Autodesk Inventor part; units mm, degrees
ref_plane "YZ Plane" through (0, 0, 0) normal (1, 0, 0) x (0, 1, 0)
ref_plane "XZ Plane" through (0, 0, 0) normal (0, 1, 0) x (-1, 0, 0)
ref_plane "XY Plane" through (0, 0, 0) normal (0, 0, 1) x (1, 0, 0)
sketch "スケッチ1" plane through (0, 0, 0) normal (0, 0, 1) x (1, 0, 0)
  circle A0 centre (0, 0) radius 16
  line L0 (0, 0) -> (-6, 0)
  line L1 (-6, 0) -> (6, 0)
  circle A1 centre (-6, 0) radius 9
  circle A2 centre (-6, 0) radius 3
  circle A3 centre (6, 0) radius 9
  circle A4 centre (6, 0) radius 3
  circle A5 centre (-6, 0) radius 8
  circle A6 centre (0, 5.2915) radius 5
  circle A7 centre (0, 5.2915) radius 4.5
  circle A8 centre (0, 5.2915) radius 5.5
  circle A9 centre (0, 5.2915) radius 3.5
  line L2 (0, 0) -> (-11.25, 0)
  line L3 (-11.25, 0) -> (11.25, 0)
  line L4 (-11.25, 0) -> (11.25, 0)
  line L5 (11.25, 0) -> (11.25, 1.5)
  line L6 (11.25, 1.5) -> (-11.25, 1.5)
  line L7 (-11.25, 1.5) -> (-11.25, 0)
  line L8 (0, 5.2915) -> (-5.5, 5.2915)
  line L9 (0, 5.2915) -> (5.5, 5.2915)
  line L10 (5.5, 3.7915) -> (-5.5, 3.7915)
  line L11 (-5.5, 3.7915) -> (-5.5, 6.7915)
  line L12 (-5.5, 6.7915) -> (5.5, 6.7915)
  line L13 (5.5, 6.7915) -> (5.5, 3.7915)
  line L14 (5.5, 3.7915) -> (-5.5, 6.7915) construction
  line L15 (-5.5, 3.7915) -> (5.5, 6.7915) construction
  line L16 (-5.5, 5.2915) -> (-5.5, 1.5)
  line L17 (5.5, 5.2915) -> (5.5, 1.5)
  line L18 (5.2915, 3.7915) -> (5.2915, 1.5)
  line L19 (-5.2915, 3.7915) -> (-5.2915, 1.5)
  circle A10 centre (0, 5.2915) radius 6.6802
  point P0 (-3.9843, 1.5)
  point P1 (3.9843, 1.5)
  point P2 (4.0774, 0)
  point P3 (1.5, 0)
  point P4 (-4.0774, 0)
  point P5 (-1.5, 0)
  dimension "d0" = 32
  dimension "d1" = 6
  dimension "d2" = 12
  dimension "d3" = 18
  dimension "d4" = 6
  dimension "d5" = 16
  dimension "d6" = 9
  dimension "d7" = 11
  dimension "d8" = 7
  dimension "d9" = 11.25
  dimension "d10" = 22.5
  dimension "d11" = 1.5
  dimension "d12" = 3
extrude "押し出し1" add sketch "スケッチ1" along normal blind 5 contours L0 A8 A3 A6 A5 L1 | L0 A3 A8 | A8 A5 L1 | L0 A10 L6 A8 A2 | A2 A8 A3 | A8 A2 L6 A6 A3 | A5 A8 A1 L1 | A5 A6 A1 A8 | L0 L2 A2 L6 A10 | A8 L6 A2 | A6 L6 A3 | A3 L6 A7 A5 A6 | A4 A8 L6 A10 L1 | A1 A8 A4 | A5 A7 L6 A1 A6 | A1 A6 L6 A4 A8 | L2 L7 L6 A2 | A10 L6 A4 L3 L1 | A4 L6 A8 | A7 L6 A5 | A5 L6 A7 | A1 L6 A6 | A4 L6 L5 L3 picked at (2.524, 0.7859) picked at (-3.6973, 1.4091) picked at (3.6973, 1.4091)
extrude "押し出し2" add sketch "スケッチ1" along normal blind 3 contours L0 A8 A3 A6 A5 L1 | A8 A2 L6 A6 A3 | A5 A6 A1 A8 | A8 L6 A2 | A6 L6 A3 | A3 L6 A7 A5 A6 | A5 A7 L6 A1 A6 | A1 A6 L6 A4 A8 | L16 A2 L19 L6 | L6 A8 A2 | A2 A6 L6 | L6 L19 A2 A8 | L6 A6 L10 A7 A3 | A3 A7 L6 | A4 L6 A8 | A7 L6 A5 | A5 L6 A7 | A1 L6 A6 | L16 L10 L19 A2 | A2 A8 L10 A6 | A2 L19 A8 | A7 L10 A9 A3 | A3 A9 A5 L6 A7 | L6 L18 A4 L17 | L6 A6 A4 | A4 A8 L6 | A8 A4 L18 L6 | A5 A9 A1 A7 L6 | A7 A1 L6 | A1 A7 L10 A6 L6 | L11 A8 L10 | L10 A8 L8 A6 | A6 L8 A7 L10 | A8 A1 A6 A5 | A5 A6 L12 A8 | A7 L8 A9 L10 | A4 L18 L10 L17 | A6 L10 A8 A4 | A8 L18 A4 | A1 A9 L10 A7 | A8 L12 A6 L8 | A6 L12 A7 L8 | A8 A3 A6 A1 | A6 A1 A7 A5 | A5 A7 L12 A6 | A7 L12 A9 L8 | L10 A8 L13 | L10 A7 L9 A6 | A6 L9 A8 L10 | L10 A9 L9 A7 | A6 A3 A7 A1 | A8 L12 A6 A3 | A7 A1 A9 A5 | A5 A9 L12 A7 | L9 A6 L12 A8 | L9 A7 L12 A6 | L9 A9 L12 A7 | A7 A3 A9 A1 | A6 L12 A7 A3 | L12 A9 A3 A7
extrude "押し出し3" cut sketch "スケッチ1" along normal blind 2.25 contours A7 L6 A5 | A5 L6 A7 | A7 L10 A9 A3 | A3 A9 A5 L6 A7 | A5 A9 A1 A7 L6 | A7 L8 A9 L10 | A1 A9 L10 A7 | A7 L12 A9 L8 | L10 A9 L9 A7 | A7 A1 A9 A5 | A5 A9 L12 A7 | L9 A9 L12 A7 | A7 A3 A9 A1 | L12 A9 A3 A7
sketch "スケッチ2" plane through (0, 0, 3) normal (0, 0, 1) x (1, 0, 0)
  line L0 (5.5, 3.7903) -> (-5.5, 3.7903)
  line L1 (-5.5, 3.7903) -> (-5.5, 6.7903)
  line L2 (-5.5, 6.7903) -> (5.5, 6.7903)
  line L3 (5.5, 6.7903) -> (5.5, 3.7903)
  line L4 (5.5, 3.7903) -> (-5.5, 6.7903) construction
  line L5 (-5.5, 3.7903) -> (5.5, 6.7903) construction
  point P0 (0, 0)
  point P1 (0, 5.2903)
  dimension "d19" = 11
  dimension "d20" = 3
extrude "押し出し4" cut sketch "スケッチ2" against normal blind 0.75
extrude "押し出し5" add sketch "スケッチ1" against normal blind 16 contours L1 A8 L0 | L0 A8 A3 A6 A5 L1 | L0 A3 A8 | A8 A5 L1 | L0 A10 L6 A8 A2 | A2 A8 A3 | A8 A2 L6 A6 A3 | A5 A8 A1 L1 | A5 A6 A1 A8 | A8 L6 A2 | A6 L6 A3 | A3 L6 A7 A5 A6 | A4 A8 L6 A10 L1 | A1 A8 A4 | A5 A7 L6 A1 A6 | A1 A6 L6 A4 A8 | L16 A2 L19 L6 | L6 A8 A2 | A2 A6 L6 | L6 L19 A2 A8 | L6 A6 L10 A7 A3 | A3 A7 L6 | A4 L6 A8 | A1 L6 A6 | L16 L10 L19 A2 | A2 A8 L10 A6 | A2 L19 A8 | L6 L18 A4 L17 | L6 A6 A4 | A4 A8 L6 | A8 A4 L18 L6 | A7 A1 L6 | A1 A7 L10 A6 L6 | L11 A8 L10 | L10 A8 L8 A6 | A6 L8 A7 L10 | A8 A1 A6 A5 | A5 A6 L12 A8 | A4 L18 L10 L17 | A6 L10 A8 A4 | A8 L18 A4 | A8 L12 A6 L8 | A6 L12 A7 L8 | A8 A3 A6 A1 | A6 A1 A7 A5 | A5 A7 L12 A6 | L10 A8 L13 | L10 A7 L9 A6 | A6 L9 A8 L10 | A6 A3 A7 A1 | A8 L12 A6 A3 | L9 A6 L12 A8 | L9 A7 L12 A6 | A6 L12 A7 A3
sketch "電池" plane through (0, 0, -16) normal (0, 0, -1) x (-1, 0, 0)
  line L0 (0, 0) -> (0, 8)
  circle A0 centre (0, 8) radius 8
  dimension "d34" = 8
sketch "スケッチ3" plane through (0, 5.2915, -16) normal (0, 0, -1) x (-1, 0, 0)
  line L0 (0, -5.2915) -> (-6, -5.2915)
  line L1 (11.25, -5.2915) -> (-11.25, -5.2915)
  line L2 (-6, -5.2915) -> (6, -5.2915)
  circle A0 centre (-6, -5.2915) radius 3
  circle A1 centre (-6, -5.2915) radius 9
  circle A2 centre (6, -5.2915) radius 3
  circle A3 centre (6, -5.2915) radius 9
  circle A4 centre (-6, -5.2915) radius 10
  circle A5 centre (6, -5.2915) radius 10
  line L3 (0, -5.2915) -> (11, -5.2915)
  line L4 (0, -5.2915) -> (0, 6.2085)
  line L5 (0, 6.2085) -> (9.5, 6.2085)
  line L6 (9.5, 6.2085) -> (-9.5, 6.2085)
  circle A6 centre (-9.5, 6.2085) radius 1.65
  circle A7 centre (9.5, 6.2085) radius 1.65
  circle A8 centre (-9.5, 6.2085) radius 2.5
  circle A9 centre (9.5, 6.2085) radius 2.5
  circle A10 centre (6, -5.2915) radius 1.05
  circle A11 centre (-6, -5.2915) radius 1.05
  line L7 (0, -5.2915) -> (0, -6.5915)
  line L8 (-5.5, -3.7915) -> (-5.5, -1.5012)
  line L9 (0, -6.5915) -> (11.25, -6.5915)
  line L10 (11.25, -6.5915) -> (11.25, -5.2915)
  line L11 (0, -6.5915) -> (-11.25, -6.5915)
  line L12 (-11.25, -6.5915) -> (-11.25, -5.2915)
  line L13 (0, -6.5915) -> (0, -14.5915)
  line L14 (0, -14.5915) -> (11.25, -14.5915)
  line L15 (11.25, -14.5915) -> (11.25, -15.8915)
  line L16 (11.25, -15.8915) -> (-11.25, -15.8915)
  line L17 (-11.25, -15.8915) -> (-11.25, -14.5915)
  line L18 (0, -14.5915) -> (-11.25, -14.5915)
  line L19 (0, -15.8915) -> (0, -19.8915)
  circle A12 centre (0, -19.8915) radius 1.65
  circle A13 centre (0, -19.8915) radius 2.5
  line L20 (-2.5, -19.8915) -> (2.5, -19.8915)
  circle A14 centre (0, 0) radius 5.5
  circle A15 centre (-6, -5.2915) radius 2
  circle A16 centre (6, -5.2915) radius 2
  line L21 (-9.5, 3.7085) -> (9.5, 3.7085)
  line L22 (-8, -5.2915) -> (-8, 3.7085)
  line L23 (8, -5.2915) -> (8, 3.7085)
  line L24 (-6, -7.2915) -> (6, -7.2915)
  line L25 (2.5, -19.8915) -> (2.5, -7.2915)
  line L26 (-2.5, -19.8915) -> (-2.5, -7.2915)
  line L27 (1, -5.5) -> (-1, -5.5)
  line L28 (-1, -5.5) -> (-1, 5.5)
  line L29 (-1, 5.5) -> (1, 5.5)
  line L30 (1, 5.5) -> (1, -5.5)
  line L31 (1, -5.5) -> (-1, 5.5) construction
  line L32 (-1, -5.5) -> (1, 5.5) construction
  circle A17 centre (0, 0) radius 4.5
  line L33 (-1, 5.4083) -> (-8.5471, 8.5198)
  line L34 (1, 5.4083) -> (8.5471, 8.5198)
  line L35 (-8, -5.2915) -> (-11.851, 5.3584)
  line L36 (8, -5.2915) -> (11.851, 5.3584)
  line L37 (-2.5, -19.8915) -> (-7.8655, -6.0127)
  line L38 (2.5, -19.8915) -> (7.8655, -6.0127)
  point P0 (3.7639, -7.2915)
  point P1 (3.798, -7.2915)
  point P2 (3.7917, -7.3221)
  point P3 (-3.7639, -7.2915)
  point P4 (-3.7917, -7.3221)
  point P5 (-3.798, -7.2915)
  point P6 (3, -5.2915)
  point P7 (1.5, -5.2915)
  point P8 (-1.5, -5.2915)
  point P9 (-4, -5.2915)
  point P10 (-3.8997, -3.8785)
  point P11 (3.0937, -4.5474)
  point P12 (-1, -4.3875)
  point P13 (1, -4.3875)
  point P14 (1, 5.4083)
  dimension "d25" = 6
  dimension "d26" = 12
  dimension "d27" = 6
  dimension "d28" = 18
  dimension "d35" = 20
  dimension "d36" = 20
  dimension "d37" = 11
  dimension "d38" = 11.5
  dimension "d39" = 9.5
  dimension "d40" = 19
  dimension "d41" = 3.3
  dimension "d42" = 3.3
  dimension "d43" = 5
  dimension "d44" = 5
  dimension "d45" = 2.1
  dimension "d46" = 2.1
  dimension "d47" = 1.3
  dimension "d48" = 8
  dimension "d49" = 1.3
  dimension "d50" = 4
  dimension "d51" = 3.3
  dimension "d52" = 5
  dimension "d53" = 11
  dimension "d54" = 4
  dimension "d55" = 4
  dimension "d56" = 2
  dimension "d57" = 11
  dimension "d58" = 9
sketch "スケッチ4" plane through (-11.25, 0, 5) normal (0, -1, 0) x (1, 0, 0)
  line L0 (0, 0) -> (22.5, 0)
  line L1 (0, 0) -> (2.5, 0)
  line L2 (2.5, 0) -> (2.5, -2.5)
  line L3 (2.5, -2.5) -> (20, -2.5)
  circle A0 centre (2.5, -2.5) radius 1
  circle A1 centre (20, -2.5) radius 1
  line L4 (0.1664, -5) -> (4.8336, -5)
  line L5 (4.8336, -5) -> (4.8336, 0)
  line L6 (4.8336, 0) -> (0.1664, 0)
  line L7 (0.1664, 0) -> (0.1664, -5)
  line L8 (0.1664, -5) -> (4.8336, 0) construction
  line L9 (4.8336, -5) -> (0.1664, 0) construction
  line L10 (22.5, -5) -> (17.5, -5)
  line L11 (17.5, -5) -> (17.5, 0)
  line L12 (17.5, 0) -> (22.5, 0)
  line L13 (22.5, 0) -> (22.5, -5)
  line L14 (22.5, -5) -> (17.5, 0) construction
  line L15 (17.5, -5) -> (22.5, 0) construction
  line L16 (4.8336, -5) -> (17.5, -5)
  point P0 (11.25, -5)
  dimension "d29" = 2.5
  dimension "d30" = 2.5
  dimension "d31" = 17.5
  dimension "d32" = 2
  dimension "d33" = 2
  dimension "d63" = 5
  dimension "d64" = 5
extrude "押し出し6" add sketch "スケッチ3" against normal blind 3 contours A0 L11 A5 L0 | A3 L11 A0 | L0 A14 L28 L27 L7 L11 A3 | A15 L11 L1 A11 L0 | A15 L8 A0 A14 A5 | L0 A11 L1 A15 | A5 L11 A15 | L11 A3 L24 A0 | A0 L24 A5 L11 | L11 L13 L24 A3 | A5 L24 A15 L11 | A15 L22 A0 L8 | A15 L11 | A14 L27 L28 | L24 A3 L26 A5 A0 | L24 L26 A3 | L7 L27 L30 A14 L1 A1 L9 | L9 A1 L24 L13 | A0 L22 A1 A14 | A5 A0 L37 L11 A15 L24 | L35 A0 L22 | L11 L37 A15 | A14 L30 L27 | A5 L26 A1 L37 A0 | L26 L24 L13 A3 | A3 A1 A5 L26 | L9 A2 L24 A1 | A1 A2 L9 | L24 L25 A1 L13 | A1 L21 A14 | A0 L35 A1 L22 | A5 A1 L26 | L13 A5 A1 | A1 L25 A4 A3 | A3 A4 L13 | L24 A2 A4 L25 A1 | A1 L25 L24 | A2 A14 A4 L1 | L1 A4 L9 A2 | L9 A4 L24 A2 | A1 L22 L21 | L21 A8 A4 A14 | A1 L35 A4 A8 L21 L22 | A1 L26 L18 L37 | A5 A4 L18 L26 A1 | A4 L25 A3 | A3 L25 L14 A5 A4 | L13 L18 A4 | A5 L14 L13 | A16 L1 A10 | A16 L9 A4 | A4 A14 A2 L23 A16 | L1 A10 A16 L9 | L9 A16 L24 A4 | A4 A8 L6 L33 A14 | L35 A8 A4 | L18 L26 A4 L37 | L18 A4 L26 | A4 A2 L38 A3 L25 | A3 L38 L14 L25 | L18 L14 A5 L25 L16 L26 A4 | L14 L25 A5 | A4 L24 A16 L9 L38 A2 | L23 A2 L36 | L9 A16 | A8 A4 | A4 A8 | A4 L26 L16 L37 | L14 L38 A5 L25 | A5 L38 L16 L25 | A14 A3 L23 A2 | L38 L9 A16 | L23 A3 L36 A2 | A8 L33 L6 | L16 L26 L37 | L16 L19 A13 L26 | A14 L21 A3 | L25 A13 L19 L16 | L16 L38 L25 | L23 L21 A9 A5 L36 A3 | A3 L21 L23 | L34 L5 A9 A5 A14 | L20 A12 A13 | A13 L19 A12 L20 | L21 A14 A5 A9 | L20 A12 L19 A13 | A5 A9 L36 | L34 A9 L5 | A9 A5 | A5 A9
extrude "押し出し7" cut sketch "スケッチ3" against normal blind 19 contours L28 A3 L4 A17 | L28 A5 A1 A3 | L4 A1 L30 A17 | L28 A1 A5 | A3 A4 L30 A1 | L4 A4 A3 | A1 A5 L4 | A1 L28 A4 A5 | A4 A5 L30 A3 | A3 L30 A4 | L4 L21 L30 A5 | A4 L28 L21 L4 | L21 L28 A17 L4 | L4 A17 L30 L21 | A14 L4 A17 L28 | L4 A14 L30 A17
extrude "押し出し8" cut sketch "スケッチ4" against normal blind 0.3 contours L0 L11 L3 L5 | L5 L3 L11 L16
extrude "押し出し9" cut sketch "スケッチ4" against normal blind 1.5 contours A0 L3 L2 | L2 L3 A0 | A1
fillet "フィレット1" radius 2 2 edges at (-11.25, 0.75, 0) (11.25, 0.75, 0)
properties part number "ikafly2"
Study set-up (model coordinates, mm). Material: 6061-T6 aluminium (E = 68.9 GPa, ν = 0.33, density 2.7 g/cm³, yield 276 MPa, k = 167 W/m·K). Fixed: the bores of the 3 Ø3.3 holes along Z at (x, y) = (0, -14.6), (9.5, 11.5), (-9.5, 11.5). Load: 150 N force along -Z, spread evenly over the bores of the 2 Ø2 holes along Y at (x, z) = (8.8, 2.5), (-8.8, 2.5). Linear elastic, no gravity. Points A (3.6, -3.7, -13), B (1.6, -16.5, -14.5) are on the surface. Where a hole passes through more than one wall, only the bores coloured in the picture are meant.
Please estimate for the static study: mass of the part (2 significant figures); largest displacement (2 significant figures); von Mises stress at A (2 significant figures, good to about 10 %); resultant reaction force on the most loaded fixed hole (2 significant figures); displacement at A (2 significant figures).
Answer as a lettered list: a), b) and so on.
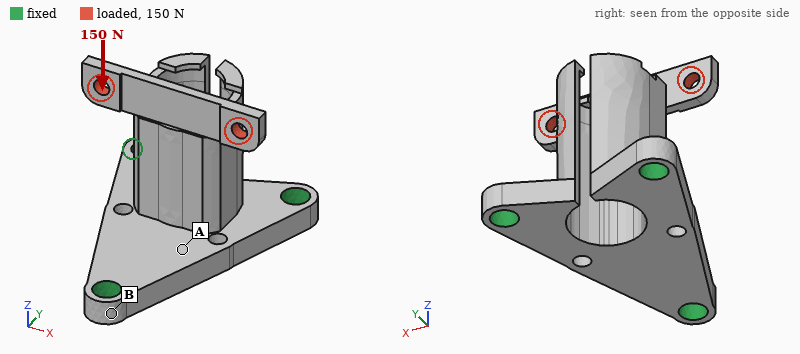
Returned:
a) 4.6 g
b) 30 µm
c) 11 MPa
d) 55 N
e) 6.6 µm
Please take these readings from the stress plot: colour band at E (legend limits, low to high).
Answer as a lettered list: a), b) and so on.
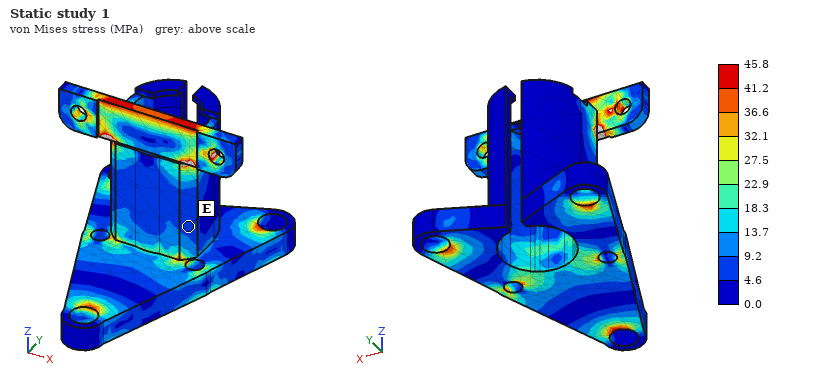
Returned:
a) 4.6 to 9.2 MPa
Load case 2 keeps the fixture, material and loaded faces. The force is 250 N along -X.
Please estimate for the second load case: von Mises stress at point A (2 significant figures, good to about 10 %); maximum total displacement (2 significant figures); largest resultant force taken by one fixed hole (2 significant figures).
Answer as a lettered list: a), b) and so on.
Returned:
a) 15 MPa
b) 0.11 mm
c) 260 N
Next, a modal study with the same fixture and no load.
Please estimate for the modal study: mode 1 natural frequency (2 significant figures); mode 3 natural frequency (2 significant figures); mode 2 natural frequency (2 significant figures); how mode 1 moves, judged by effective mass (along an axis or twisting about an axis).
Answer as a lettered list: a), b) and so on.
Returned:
a) 7700 Hz
b) 11 kHz
c) 8400 Hz
d) along X
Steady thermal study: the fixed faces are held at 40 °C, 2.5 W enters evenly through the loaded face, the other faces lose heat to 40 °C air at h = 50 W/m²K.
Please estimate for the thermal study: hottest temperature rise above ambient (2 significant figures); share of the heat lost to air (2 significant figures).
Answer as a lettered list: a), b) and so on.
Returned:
a) 14 K
b) 15 %
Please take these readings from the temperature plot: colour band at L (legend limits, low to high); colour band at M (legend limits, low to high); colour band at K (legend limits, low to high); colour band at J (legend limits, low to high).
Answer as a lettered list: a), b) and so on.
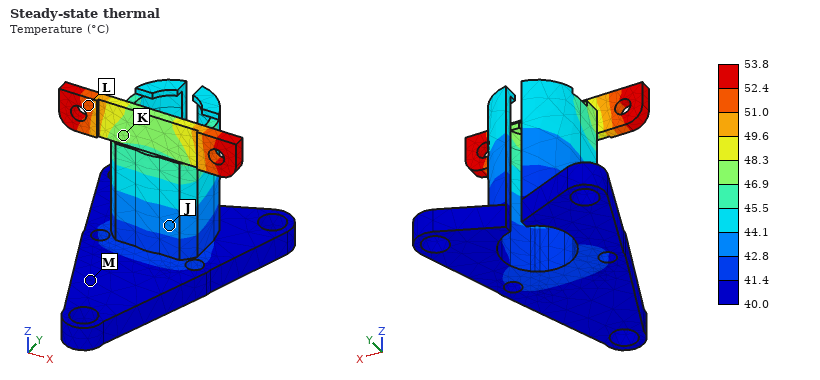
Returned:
a) 51.0 to 52.4 °C
b) 40.0 to 41.4 °C
c) 46.9 to 48.3 °C
d) 42.8 to 44.1 °C
